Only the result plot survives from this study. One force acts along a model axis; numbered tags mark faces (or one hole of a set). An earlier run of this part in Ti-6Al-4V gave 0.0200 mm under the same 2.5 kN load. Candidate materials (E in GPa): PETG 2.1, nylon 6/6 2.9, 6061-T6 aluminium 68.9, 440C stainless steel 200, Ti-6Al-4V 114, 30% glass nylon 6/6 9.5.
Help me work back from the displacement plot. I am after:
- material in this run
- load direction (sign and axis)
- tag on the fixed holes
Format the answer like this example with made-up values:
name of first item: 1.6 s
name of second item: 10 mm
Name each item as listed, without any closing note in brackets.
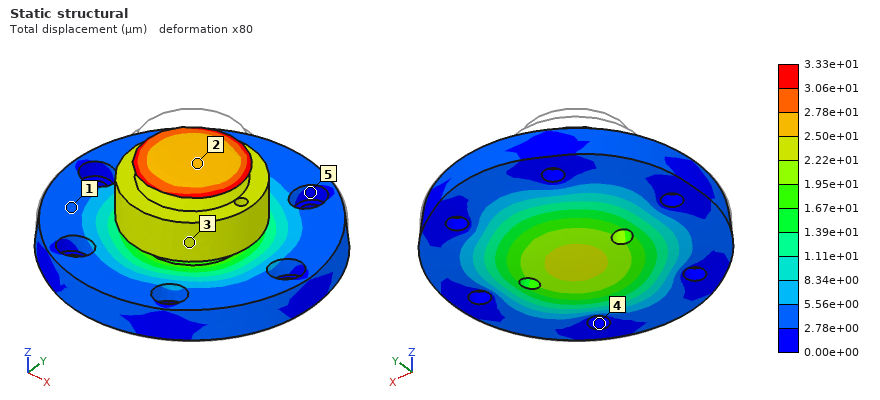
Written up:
material in this run: 6061-T6 aluminium
load direction: -Z
tag on the fixed holes: 4
